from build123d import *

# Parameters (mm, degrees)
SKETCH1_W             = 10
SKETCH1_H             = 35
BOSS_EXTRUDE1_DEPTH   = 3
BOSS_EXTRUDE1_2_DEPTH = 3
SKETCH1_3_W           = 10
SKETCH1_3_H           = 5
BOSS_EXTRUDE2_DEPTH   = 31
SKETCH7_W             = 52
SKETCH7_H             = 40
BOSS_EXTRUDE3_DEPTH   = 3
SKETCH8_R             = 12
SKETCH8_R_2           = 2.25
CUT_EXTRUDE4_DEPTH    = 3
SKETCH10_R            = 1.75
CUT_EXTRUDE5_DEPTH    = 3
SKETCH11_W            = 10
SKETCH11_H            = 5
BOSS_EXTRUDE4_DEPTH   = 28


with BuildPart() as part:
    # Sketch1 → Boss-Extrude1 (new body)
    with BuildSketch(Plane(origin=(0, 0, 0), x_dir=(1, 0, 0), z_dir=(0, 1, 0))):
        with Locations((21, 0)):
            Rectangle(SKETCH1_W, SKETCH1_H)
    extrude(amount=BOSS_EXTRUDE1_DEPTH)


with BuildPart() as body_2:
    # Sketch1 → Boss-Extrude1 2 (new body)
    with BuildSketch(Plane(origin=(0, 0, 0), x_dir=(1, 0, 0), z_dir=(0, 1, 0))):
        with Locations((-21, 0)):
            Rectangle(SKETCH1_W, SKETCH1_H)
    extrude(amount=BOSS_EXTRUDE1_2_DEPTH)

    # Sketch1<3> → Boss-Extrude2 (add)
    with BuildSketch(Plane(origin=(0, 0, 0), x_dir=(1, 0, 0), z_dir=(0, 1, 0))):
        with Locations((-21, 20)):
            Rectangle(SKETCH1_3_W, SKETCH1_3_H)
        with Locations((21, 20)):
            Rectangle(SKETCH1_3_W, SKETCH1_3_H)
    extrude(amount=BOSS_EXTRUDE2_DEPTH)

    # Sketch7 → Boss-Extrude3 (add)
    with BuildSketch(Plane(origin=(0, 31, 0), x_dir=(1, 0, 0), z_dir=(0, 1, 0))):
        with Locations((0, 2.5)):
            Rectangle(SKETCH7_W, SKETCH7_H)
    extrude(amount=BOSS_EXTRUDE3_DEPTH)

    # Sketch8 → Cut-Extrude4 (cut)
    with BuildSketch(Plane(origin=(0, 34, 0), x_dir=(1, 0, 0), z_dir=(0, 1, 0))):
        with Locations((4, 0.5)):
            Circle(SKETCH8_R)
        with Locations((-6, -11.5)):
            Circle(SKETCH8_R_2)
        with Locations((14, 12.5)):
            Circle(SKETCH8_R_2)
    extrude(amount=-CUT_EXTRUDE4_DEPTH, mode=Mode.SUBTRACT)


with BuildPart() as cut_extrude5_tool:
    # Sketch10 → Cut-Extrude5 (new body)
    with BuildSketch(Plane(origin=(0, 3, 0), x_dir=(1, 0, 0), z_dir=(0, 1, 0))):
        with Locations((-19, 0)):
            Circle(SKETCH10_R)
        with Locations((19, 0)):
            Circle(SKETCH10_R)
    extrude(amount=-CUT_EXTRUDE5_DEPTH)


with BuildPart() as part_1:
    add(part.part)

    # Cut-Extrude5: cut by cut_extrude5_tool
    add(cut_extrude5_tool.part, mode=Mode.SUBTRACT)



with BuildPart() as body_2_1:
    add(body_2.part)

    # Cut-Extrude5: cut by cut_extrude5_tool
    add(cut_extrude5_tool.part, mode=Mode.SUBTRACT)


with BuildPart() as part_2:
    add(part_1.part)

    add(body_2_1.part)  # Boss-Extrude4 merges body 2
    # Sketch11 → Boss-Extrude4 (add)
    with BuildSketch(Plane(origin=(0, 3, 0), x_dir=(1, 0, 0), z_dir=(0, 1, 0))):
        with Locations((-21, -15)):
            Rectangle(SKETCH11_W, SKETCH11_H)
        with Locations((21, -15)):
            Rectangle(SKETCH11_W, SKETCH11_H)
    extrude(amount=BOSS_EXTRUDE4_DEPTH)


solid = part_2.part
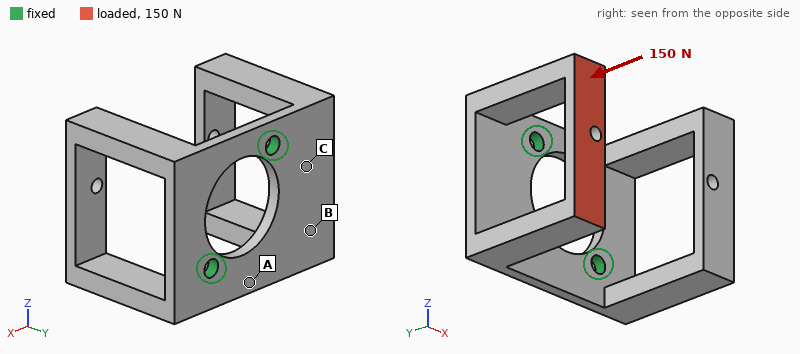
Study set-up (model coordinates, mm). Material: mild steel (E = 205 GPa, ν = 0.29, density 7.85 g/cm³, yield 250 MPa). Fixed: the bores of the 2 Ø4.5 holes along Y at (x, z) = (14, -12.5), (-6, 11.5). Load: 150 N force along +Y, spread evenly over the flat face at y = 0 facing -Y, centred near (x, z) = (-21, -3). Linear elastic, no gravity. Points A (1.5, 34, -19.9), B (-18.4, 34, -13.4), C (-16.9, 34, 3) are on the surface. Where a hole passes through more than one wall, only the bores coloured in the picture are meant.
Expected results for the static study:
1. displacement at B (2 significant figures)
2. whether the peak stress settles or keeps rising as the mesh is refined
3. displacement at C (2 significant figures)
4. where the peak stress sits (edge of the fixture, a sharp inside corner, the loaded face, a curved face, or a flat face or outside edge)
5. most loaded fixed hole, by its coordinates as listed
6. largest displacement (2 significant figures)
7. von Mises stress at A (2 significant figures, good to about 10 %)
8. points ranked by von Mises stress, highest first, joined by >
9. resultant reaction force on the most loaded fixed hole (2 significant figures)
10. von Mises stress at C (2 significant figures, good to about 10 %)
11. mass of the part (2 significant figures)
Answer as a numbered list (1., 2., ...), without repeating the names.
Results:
1. 0.045 mm
2. keeps rising
3. 0.019 mm
4. edge of the fixture
5. (-6, 11.5)
6. 0.11 mm
7. 33 MPa
8. A > C > B
9. 130 N
10. 17 MPa
11. 100 g
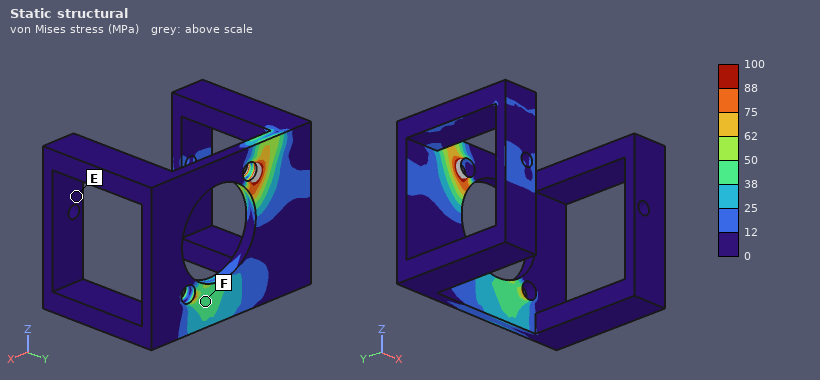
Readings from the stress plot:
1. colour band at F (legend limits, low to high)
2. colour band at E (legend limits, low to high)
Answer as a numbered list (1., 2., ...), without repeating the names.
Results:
1. 38 to 50 MPa
2. 0 to 12 MPa
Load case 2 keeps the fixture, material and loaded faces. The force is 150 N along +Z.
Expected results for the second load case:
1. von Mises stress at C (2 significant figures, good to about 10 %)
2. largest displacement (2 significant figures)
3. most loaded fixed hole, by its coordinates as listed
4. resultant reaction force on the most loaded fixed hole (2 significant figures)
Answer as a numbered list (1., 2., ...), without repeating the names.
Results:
1. 19 MPa
2. 0.15 mm
3. (-6, 11.5)
4. 170 N
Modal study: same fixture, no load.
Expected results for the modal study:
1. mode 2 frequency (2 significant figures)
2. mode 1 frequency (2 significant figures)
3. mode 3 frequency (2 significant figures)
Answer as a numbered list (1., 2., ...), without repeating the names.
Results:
1. 1400 Hz
2. 910 Hz
3. 1500 Hz
